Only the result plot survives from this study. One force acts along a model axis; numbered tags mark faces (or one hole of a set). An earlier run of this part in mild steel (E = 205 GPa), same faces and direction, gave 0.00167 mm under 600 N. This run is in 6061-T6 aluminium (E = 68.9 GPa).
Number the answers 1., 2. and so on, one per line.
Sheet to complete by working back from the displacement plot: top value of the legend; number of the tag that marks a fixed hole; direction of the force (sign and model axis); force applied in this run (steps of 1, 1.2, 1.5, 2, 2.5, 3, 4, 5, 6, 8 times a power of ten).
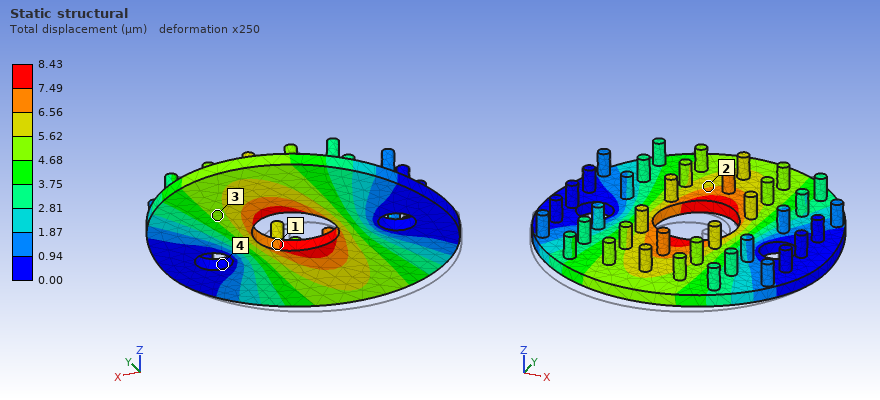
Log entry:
1. 8.43 µm
2. 4
3. +Y
4. 1 kN
